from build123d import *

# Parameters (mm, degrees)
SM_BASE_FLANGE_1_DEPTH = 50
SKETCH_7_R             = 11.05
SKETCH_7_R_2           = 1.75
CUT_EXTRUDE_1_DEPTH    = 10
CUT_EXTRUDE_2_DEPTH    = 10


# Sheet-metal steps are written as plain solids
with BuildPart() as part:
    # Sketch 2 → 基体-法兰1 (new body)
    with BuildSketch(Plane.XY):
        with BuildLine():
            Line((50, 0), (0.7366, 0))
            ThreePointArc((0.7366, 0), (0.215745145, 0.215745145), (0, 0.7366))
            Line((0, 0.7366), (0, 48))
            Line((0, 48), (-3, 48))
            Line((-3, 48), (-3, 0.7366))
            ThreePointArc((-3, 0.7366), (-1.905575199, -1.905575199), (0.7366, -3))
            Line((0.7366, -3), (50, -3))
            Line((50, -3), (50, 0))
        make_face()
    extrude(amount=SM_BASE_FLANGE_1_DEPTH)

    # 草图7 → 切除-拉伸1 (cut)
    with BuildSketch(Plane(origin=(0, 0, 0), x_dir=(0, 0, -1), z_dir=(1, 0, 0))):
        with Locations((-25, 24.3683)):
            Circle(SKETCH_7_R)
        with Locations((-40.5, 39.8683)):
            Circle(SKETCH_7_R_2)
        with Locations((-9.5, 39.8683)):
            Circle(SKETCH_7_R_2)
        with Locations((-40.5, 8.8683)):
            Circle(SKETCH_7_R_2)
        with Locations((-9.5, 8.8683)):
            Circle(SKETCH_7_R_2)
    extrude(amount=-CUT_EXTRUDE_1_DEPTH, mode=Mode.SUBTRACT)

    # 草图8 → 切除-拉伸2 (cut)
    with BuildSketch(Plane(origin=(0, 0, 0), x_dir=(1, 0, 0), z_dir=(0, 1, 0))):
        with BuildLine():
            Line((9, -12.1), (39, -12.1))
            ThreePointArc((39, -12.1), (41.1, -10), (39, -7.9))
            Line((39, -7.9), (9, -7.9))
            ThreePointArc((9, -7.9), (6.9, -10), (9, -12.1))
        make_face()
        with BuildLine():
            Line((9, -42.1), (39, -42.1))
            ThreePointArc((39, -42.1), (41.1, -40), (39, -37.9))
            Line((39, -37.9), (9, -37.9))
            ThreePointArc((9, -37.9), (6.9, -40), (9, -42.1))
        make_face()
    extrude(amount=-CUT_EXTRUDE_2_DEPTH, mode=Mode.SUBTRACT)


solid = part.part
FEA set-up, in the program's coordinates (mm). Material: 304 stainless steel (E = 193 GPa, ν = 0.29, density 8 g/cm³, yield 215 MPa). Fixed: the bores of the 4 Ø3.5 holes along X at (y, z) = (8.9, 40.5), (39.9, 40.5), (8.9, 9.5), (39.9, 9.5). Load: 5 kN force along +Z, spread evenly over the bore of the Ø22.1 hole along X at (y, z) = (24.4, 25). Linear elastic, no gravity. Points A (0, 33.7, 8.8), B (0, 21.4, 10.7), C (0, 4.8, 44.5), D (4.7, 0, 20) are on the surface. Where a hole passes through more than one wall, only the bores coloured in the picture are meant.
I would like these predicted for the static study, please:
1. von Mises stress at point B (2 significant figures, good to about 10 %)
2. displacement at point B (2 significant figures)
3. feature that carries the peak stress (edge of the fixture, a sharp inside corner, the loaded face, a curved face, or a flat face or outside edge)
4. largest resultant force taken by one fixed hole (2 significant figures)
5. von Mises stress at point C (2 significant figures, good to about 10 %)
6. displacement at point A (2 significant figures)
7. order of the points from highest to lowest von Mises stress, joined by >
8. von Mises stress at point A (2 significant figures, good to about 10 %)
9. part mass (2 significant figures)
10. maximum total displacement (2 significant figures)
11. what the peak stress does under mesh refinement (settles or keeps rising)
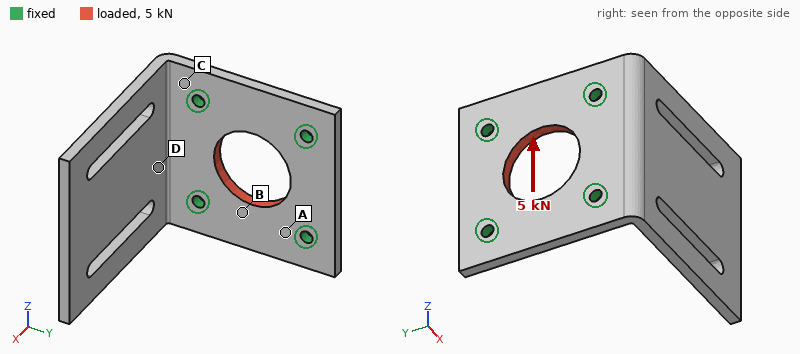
21 MPa
3.4 µm
edge of the fixture
1.3 kN
11 MPa
1.9 µm
A > B > C > D
26 MPa
100 g
4.0 µm
keeps rising
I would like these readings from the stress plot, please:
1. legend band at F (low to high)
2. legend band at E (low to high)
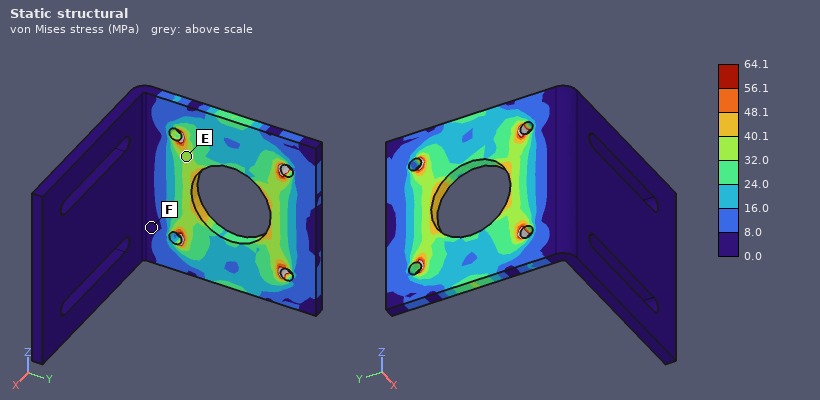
0.0 to 8.0 MPa
32.0 to 40.1 MPa
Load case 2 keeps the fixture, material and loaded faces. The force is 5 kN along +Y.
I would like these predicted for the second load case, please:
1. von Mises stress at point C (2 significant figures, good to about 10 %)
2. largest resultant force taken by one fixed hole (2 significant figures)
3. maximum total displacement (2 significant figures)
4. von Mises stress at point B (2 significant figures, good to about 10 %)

7.7 MPa
1.3 kN
4.4 µm
29 MPa
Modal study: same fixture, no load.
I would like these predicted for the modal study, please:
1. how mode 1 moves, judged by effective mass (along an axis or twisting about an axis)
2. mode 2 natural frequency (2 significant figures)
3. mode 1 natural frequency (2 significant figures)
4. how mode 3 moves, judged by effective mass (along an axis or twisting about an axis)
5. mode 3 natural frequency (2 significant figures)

along Y
1900 Hz
680 Hz
along Z
2900 Hz
